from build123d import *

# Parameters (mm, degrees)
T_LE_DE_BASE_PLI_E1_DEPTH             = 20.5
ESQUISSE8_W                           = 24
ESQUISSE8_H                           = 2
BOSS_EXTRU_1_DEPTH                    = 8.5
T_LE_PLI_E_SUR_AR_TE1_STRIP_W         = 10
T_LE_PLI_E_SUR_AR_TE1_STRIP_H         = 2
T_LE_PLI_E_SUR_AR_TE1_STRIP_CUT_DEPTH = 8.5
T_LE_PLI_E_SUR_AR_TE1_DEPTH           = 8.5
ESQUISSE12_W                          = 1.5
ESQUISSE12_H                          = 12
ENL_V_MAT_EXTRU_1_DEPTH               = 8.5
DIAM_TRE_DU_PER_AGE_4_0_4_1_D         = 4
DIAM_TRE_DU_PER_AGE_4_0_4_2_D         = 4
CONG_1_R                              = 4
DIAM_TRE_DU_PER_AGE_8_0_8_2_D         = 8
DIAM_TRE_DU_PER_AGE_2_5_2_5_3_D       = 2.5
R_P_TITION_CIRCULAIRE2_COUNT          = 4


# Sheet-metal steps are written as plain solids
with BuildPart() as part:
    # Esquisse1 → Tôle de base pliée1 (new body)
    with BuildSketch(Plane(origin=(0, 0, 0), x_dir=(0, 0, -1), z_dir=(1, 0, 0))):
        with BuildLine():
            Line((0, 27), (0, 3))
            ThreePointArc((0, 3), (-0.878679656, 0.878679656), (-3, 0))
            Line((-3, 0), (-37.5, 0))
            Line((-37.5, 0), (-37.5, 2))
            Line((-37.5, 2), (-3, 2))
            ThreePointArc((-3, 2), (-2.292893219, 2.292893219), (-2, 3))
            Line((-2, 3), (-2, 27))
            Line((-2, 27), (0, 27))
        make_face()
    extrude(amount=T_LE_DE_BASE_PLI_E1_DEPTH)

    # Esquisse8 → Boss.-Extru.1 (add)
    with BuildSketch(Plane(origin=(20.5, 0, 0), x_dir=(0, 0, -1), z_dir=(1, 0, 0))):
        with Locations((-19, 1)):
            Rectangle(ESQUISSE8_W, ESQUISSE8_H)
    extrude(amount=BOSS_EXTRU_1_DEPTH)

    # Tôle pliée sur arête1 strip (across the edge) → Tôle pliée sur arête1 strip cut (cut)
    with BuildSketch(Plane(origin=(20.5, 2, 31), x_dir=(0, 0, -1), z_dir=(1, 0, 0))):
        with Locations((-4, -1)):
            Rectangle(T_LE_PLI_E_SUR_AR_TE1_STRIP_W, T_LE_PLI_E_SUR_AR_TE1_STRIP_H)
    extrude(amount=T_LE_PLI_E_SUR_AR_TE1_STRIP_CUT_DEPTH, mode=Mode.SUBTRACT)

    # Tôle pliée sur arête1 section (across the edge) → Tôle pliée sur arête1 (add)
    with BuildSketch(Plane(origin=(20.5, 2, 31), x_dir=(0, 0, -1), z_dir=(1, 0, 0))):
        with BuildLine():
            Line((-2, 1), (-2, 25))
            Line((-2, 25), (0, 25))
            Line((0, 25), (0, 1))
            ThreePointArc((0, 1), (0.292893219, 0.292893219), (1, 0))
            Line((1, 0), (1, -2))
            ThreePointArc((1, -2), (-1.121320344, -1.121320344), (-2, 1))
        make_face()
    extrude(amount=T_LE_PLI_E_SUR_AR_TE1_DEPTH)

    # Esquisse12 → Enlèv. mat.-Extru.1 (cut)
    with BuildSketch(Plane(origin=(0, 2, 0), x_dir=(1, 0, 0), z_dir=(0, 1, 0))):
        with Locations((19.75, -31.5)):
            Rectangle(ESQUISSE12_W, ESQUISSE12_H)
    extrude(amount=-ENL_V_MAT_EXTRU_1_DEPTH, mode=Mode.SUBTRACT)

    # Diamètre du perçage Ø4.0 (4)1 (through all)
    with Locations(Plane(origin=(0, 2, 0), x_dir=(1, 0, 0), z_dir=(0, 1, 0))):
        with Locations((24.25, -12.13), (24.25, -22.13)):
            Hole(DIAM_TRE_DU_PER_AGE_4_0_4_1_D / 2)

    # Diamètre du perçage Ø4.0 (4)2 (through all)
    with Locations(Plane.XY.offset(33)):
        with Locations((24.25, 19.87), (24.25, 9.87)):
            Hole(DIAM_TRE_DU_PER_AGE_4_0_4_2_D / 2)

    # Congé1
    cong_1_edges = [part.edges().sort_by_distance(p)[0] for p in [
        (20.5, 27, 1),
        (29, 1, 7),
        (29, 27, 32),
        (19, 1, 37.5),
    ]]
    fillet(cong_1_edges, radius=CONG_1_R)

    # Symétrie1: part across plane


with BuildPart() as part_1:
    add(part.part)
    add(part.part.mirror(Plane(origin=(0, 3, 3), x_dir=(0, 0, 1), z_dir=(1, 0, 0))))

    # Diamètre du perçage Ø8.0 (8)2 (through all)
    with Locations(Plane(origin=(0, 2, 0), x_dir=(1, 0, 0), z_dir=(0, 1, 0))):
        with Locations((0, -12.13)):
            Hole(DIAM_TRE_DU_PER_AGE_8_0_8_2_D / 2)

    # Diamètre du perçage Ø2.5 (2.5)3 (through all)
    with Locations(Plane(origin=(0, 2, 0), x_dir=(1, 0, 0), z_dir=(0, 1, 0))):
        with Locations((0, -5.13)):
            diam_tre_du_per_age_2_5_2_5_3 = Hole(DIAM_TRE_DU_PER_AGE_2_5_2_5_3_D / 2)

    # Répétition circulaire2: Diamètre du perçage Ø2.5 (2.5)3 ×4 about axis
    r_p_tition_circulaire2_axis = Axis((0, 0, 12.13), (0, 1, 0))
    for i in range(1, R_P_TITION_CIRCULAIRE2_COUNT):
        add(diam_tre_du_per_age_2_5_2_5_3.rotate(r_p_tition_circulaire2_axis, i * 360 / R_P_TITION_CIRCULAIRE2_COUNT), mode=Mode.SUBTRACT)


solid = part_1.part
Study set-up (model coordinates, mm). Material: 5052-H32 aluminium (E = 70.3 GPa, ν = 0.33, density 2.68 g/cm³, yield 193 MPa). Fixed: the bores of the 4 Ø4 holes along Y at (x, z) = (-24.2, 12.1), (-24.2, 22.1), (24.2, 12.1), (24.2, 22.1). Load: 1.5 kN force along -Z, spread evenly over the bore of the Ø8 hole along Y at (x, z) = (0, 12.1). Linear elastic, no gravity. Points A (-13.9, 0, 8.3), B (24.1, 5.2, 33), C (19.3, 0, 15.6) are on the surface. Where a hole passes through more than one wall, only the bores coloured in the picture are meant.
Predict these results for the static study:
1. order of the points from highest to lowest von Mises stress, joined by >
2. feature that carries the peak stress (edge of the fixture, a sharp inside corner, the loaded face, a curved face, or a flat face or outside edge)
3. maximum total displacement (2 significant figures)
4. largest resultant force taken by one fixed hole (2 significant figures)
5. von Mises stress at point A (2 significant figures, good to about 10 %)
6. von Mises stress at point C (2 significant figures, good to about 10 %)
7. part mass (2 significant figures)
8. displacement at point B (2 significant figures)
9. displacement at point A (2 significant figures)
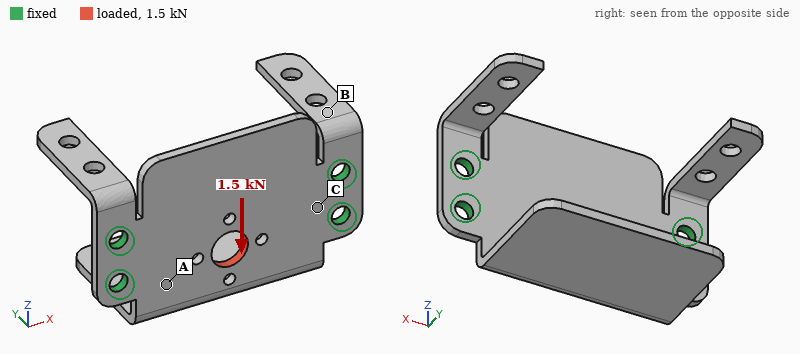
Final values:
C > A > B
a curved face
20 µm
460 N
19 MPa
37 MPa
17 g
3.5 µm
8.0 µm
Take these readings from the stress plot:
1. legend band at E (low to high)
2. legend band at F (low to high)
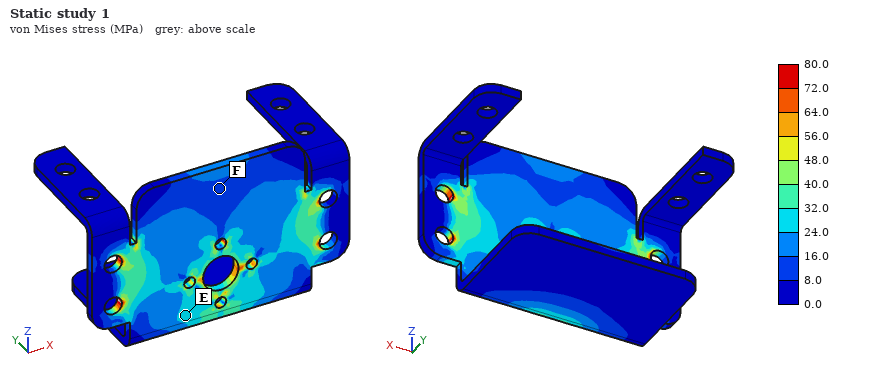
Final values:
24.0 to 32.0 MPa
8.0 to 16.0 MPa
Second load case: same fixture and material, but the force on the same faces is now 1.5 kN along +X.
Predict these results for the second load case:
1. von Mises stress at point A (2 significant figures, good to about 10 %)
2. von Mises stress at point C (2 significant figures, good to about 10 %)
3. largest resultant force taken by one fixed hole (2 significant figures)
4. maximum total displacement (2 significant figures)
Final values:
24 MPa
16 MPa
470 N
8.9 µm
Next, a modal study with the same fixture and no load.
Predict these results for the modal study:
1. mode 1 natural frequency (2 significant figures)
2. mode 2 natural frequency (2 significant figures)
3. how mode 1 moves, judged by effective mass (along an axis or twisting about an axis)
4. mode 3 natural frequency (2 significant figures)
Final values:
1300 Hz
1700 Hz
along Z
1700 Hz
